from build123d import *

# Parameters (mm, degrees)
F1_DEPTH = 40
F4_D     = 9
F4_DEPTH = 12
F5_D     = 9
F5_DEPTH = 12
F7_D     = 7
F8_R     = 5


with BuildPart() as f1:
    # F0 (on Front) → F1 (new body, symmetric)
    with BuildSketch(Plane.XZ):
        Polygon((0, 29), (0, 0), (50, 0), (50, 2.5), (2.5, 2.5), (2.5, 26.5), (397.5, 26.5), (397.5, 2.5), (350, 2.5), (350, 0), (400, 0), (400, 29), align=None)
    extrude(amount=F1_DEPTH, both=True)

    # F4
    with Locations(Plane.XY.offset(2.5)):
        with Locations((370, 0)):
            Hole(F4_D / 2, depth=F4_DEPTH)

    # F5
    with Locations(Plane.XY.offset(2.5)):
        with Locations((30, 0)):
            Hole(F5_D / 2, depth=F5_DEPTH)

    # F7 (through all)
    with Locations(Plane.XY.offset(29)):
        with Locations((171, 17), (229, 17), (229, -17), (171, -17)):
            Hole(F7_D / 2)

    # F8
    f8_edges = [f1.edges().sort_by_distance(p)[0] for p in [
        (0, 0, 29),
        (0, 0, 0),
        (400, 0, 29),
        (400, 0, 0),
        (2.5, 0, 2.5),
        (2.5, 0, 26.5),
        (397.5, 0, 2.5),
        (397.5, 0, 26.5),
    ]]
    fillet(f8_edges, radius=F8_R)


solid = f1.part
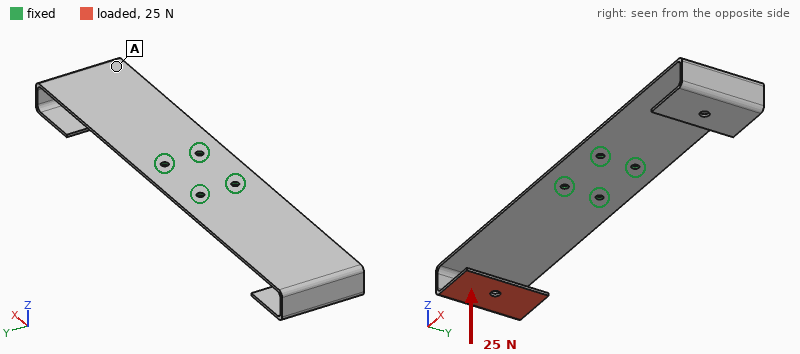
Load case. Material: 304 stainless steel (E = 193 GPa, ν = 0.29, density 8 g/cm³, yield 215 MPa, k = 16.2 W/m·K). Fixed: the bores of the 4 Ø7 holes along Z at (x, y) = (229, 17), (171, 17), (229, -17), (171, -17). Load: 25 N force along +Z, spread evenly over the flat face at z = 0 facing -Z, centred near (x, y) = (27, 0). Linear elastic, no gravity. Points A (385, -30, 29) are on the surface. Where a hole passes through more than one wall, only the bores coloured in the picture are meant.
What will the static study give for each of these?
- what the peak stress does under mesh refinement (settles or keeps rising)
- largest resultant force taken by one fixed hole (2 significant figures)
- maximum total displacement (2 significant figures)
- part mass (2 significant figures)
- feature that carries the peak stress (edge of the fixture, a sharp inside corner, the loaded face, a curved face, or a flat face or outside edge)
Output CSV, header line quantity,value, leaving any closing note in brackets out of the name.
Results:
quantity,value
what the peak stress does under mesh refinement,keeps rising
largest resultant force taken by one fixed hole,16 N
maximum total displacement,1.5 mm
part mass,870 g
feature that carries the peak stress,edge of the fixture
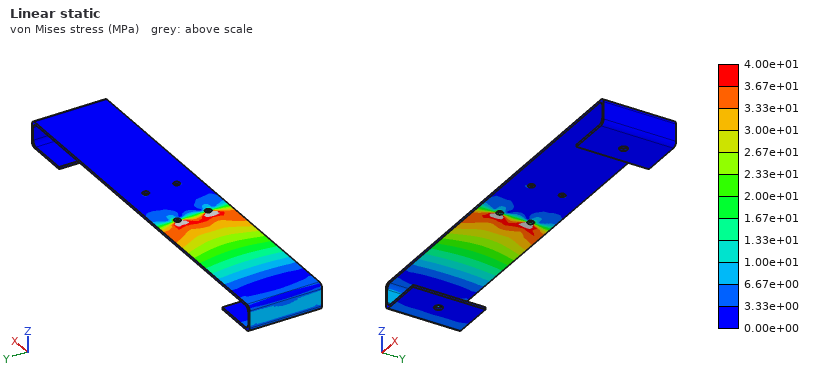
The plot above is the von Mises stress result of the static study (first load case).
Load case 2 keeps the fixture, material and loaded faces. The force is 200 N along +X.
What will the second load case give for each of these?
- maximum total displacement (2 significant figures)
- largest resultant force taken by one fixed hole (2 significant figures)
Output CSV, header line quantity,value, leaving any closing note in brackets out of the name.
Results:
quantity,value
maximum total displacement,4.1 mm
largest resultant force taken by one fixed hole,87 N
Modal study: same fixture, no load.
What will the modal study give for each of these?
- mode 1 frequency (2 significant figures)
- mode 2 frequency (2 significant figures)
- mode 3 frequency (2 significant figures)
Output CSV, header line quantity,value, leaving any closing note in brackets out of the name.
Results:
quantity,value
mode 1 frequency,45 Hz
mode 2 frequency,45 Hz
mode 3 frequency,170 Hz
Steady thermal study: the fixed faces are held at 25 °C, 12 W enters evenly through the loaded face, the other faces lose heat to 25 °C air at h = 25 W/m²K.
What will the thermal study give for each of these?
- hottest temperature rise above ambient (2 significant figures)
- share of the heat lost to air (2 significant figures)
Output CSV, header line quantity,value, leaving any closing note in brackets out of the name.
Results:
quantity,value
hottest temperature rise above ambient,76 K
share of the heat lost to air,100 %
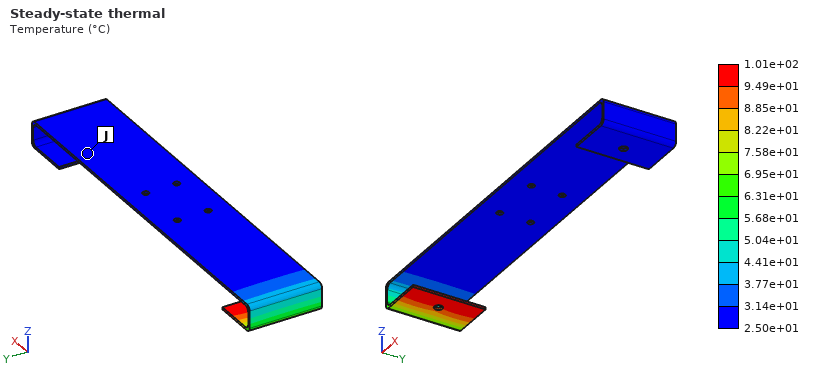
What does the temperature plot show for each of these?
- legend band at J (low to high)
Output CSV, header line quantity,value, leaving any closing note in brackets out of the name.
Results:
quantity,value
legend band at J,2.50e+01 to 3.14e+01 °C
